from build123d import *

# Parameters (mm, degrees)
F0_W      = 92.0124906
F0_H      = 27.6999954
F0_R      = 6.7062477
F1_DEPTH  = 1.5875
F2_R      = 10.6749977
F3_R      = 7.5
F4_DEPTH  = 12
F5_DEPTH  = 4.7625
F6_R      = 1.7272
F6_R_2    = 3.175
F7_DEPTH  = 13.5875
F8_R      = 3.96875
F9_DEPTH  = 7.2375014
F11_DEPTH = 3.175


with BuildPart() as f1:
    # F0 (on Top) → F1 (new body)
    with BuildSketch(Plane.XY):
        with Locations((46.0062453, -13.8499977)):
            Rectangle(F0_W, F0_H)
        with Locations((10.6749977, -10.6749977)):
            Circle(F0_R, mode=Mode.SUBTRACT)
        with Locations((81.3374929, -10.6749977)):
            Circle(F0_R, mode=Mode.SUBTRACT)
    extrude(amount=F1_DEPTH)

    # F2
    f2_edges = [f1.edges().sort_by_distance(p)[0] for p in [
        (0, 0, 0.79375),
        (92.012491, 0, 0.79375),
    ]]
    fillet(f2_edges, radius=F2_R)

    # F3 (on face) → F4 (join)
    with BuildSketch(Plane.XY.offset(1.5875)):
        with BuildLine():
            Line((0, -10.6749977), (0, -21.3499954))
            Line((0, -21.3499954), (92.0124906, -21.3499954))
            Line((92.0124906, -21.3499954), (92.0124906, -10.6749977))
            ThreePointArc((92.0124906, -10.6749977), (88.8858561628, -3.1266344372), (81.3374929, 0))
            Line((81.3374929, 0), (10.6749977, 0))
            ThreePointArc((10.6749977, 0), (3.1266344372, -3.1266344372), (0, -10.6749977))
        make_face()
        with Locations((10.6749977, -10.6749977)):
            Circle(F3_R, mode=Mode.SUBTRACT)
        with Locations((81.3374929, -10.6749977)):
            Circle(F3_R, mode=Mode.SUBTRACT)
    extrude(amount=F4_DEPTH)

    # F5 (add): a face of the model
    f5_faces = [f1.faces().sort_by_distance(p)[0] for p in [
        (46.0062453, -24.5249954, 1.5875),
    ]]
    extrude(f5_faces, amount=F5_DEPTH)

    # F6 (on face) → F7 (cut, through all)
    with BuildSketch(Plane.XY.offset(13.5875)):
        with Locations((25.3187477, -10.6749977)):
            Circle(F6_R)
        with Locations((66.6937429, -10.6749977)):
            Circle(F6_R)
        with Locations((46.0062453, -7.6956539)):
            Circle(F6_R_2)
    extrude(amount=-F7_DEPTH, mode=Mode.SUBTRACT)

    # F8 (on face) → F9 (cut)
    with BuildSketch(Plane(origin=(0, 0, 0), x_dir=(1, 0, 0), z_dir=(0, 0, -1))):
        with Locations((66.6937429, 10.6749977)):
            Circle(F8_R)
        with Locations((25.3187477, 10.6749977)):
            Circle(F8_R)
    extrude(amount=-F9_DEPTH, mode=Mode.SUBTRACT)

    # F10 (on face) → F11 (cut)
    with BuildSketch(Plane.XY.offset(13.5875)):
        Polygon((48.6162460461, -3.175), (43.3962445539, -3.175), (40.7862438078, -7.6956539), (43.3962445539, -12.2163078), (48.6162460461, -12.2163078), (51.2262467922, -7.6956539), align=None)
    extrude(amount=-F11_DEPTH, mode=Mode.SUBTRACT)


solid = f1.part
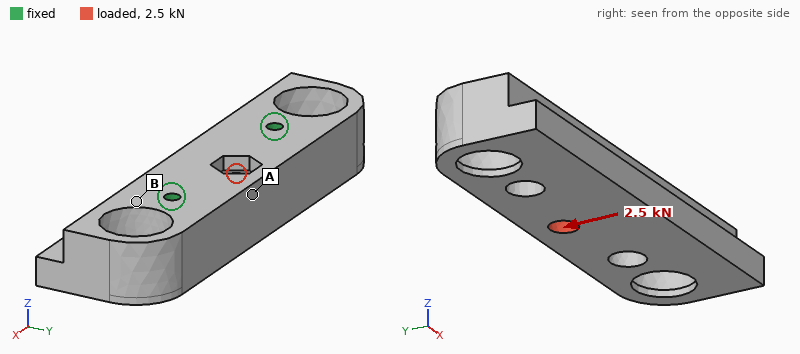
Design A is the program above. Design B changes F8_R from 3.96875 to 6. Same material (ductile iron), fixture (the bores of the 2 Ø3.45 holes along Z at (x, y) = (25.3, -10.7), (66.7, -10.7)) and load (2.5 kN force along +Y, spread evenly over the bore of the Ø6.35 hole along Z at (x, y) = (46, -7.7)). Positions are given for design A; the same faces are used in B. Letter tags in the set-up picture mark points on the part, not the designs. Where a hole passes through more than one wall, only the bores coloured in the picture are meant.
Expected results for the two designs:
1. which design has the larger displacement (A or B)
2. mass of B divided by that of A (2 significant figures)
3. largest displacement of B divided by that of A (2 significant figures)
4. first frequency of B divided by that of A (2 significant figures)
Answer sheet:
B
0.96
1.1
0.96
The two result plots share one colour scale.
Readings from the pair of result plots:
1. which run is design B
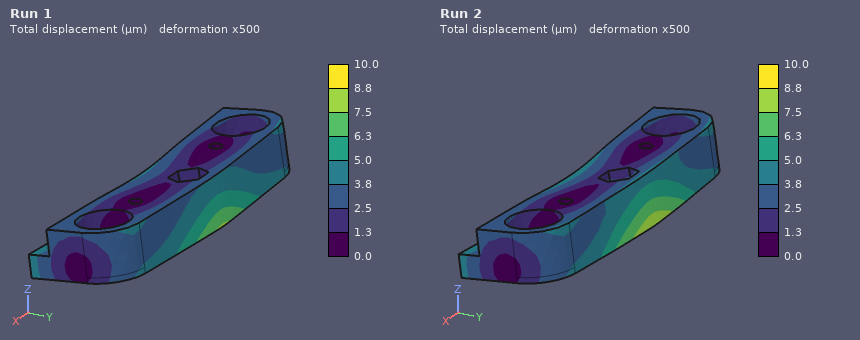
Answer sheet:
Run 2
